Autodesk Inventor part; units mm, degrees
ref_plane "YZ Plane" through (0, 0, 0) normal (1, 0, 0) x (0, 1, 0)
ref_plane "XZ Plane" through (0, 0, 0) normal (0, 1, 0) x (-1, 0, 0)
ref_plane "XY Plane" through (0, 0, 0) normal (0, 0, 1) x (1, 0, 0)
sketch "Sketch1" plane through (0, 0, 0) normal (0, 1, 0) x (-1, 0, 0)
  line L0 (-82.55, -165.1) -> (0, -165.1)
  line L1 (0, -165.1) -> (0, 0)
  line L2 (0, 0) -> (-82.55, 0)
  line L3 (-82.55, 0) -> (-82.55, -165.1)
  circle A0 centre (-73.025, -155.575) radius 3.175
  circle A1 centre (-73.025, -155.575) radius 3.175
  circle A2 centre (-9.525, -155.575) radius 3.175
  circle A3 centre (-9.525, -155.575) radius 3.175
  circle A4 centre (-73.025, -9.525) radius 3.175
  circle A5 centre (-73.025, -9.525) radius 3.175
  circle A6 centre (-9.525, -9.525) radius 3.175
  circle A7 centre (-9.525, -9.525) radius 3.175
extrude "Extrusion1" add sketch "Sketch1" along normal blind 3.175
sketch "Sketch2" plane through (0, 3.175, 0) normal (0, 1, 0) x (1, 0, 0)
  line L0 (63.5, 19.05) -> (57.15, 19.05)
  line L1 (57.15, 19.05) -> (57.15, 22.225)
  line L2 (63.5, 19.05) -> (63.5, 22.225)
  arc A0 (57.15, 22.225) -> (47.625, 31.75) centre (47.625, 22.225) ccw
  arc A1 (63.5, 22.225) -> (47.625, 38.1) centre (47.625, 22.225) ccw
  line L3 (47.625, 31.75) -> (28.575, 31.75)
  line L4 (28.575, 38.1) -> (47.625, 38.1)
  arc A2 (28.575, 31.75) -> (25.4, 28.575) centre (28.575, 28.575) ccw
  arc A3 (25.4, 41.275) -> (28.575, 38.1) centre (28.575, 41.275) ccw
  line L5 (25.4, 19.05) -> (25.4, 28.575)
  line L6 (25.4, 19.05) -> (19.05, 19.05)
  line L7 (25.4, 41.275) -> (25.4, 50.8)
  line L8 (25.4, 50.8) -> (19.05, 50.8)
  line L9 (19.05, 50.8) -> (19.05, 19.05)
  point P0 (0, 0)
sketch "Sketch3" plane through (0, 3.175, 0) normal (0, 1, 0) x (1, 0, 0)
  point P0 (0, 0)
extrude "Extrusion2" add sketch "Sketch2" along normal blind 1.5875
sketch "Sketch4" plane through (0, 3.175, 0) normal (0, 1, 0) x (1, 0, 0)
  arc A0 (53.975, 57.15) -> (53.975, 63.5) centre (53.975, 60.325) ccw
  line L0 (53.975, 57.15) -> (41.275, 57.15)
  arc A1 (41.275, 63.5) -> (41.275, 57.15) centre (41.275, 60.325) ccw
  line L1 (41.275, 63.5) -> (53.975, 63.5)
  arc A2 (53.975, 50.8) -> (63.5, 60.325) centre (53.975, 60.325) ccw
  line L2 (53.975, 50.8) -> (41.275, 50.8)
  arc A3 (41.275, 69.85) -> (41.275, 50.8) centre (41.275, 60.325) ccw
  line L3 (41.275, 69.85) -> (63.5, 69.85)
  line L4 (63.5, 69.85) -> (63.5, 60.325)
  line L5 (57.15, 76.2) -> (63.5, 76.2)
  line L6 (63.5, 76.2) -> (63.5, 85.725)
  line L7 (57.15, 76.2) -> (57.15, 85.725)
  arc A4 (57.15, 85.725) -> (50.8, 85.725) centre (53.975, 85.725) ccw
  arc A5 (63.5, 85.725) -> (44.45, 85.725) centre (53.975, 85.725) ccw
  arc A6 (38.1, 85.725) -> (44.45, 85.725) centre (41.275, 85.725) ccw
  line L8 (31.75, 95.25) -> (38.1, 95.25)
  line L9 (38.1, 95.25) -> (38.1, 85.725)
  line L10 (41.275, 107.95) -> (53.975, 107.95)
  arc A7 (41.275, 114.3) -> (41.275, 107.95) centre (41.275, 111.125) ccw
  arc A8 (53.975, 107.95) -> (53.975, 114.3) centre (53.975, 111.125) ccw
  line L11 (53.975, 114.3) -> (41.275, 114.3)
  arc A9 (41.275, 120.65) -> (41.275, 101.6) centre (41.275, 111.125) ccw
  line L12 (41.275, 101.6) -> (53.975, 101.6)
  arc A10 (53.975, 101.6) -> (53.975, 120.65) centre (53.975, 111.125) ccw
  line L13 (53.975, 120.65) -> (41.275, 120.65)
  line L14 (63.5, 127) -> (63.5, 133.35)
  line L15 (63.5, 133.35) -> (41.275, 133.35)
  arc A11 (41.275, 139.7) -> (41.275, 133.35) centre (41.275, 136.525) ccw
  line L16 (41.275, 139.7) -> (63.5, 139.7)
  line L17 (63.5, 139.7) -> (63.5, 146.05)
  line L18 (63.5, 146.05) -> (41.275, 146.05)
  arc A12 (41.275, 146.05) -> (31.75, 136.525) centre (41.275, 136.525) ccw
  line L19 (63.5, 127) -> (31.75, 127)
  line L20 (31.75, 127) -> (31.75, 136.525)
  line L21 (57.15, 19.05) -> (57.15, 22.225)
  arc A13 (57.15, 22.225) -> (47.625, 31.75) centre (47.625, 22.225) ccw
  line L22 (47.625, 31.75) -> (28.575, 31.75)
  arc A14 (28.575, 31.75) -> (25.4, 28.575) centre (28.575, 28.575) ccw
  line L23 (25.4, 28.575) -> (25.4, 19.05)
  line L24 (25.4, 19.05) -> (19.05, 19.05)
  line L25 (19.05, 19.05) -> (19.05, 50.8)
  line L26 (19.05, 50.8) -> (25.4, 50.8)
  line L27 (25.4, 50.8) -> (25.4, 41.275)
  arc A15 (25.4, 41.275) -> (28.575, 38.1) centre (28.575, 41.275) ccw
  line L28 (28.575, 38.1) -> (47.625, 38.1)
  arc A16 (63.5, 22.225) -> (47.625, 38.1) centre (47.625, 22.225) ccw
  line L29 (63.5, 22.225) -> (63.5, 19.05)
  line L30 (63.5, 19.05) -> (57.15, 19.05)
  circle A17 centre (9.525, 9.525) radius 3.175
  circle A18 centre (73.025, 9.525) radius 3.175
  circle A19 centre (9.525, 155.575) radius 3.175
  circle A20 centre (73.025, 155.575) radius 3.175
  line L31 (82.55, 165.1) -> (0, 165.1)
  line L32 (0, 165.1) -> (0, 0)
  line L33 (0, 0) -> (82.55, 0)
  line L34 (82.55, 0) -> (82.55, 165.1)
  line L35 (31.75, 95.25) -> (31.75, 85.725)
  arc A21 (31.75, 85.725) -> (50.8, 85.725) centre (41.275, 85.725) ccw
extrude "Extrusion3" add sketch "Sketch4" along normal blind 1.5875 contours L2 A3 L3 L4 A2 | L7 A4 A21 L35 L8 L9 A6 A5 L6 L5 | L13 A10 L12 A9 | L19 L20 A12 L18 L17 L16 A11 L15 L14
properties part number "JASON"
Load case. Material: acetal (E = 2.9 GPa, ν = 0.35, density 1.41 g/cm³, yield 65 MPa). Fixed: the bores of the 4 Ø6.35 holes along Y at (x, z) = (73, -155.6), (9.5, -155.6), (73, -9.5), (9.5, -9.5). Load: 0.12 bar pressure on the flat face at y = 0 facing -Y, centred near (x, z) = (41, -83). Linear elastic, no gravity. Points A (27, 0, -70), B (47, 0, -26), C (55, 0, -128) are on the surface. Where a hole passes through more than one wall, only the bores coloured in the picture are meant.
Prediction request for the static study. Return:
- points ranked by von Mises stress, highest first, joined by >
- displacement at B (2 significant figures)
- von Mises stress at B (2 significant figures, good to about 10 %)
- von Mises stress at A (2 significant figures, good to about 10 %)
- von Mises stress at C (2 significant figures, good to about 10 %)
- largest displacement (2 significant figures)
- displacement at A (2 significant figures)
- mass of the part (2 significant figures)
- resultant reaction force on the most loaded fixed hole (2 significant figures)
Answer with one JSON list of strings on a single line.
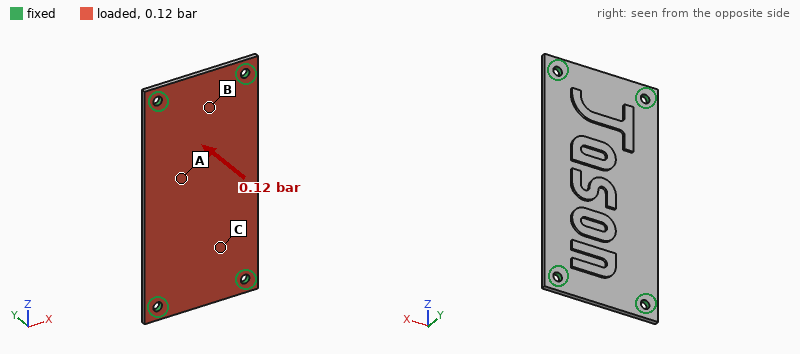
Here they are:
["A > B > C", "0.45 mm", "2.9 MPa", "5.3 MPa", "1.6 MPa", "1.9 mm", "1.7 mm", "65 g", "43 N"]
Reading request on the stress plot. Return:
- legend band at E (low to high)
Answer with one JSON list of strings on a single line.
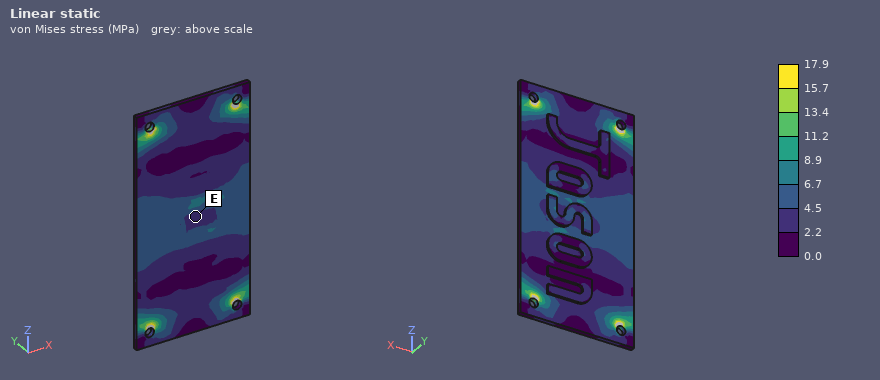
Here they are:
["2.2 to 4.5 MPa"]
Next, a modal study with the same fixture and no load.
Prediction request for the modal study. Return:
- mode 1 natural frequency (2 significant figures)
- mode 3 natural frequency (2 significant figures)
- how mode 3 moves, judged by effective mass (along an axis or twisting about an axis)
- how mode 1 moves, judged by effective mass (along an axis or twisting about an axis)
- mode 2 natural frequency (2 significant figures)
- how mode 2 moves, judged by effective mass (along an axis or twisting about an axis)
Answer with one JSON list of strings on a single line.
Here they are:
["210 Hz", "590 Hz", "twisting about X", "along Y", "370 Hz", "twisting about Z"]
